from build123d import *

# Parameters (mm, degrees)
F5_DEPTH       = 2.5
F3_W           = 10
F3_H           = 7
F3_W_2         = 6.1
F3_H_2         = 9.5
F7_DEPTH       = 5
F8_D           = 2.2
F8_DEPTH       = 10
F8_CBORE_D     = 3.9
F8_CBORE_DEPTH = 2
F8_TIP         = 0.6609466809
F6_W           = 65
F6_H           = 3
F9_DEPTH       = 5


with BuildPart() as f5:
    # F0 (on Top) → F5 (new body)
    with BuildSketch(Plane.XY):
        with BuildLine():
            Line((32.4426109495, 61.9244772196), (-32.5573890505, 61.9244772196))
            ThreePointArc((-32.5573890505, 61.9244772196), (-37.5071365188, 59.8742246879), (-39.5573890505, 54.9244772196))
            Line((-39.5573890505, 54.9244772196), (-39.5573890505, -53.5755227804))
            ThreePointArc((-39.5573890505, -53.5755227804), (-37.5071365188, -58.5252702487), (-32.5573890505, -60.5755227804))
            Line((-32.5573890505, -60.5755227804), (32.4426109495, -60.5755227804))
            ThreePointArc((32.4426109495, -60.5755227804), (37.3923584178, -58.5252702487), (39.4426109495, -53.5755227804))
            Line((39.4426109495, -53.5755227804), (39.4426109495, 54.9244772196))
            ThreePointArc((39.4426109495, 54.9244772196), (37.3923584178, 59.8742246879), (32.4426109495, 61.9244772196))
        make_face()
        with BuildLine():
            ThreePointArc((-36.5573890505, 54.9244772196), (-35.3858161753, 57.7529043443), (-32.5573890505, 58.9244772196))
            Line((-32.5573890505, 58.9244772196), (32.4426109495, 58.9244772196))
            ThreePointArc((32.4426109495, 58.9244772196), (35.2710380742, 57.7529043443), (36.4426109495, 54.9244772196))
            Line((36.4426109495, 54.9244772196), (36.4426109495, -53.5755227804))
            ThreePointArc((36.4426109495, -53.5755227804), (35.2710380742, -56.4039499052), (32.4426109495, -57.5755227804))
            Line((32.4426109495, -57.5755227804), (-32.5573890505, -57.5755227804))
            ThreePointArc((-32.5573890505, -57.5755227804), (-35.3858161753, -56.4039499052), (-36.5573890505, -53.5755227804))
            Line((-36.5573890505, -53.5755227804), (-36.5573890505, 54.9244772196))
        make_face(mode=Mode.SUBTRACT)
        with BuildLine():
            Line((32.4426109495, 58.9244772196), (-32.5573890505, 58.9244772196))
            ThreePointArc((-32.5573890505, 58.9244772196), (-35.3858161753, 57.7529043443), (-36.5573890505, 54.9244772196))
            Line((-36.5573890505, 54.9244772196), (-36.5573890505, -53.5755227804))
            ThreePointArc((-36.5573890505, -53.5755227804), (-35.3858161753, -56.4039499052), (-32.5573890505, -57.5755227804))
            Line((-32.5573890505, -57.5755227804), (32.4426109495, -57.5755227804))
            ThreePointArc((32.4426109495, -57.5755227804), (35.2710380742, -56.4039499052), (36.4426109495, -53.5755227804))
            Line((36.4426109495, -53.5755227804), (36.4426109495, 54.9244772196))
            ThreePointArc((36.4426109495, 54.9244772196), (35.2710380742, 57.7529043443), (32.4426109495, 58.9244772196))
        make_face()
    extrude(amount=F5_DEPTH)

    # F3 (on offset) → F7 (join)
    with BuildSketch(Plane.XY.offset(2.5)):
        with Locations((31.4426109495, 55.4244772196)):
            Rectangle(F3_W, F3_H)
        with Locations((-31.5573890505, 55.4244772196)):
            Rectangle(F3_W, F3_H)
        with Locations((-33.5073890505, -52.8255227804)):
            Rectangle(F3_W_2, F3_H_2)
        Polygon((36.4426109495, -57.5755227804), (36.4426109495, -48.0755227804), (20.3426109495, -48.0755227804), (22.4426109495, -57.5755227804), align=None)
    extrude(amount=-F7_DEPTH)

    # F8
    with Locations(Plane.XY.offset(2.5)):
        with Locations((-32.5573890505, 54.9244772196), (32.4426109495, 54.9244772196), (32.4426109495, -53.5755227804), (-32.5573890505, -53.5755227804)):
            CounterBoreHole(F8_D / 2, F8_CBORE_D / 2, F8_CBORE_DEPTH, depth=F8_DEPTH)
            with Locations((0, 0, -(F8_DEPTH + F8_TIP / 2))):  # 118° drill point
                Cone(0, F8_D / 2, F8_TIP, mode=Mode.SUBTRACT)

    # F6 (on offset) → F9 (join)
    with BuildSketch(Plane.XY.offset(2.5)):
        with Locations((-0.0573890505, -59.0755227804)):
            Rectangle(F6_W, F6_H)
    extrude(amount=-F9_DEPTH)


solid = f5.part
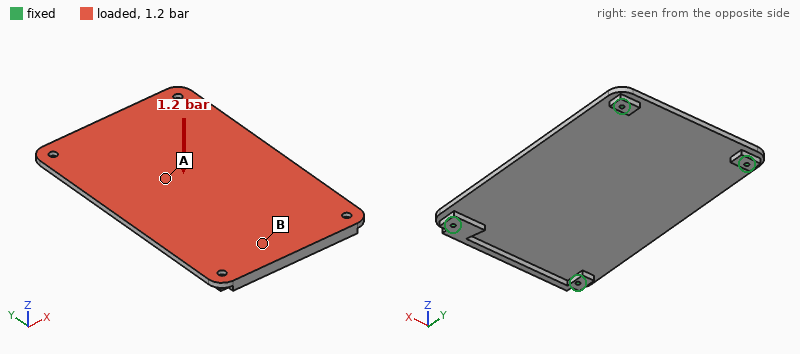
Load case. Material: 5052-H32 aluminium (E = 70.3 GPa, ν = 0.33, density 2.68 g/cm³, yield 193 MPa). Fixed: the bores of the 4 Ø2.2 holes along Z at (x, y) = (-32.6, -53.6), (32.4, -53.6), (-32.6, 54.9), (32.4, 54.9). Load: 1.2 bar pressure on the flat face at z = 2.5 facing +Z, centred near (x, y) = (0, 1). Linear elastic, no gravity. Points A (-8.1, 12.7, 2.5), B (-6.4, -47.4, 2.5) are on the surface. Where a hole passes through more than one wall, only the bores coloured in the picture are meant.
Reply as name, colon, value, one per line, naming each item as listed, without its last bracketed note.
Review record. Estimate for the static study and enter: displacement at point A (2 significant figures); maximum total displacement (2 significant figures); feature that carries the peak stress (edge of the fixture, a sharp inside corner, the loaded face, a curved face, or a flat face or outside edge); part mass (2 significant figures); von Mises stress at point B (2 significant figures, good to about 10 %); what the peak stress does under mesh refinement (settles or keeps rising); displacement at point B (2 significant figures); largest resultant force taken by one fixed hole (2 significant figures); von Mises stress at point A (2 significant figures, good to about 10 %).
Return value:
displacement at point A: 0.56 mm
maximum total displacement: 0.60 mm
feature that carries the peak stress: edge of the fixture
part mass: 68 g
von Mises stress at point B: 34 MPa
what the peak stress does under mesh refinement: keeps rising
displacement at point B: 0.12 mm
largest resultant force taken by one fixed hole: 830 N
von Mises stress at point A: 55 MPa
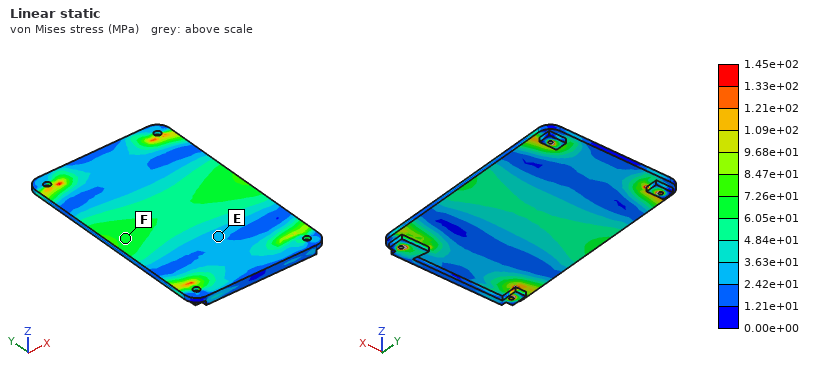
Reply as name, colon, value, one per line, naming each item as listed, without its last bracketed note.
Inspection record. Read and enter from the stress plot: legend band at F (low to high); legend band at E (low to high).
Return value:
legend band at F: 6.05e+01 to 7.26e+01 MPa
legend band at E: 2.42e+01 to 3.63e+01 MPa
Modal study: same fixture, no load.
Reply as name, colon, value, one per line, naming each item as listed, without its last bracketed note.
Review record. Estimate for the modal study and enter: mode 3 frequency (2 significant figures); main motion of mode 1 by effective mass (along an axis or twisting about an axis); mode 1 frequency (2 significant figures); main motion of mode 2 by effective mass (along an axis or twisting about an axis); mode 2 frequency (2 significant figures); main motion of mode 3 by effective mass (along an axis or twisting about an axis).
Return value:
mode 3 frequency: 2600 Hz
main motion of mode 1 by effective mass: along Z
mode 1 frequency: 1000 Hz
main motion of mode 2 by effective mass: twisting about Y
mode 2 frequency: 1500 Hz
main motion of mode 3 by effective mass: twisting about X
